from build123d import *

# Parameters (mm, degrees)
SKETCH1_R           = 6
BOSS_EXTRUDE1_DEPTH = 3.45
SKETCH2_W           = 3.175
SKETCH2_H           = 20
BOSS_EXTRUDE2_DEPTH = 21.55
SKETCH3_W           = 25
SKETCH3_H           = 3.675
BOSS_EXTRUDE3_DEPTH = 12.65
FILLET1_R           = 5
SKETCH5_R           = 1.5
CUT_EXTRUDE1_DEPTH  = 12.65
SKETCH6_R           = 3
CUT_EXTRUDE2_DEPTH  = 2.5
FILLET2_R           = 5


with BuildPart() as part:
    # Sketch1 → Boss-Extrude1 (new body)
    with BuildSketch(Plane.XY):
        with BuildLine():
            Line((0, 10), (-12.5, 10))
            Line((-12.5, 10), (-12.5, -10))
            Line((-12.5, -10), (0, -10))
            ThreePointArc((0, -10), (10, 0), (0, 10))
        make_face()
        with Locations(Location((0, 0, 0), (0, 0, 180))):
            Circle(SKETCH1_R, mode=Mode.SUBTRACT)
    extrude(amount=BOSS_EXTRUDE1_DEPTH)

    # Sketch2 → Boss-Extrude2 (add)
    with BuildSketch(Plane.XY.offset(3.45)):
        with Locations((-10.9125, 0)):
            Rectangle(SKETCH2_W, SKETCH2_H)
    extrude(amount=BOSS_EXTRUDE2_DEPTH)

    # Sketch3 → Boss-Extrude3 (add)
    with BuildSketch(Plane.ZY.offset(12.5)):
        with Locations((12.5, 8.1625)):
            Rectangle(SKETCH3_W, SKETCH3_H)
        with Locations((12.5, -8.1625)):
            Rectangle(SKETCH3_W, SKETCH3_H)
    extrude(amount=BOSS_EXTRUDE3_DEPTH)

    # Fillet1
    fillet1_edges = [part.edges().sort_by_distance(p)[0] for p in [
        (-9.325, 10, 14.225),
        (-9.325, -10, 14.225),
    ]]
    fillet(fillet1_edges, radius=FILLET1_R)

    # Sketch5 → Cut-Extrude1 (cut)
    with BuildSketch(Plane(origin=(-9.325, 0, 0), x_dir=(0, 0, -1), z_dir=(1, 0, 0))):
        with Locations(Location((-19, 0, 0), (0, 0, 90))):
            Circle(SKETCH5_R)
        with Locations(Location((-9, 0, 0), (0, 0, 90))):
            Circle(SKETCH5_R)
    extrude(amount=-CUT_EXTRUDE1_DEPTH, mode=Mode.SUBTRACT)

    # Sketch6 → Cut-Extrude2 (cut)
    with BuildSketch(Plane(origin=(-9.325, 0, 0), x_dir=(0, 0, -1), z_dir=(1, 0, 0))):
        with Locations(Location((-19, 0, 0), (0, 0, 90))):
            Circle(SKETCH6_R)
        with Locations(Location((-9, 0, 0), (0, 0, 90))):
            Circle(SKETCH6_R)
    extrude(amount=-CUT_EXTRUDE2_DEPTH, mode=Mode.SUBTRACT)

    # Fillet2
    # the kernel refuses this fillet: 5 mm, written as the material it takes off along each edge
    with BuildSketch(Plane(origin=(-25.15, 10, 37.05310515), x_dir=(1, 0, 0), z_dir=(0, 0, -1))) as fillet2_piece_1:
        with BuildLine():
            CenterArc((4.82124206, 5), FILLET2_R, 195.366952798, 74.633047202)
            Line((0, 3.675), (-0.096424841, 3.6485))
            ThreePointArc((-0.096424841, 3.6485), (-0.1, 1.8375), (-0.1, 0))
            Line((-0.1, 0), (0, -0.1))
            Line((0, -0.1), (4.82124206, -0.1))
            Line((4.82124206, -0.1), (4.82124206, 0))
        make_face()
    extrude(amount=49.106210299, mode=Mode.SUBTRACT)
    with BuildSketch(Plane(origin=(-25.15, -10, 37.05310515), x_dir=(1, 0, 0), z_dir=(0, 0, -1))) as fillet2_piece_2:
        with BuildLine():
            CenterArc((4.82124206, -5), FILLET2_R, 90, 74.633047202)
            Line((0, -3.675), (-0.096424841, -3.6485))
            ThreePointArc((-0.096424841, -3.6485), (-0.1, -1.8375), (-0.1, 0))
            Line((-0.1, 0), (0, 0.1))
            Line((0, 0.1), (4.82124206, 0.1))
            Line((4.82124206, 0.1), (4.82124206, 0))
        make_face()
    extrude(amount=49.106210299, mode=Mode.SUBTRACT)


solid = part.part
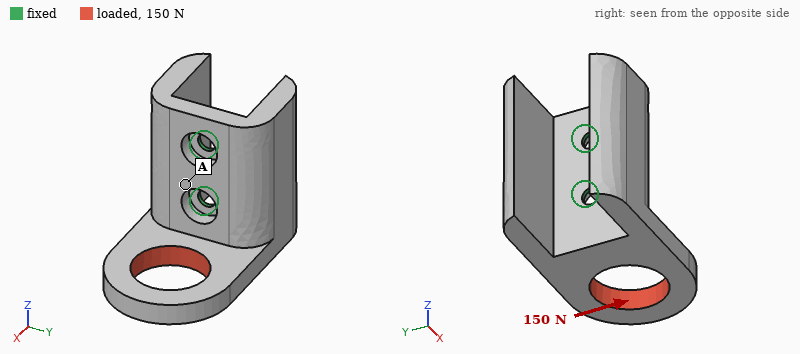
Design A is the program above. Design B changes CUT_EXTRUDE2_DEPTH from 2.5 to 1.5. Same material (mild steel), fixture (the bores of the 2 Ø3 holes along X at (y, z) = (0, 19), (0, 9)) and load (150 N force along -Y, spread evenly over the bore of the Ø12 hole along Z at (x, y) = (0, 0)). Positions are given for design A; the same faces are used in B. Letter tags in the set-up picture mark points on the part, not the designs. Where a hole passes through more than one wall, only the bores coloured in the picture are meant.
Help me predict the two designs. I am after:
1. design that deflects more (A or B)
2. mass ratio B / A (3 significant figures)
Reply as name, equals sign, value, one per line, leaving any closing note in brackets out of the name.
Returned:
design that deflects more = A
mass ratio B / A = 1.01
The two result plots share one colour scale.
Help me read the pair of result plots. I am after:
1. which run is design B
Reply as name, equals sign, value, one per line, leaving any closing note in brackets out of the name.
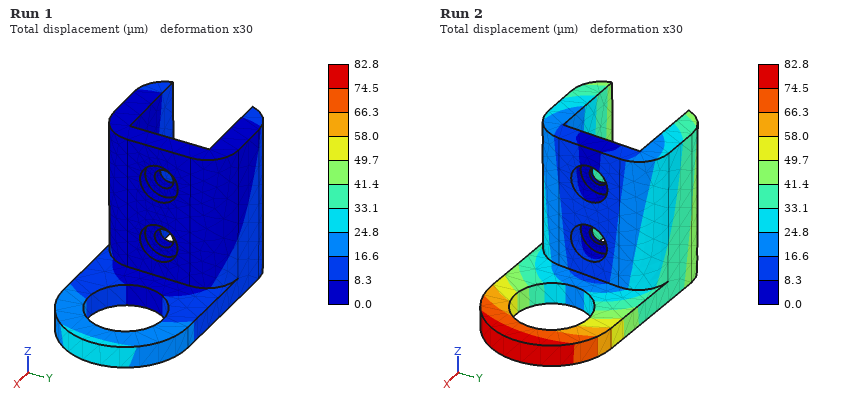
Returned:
which run is design B = Run 1
